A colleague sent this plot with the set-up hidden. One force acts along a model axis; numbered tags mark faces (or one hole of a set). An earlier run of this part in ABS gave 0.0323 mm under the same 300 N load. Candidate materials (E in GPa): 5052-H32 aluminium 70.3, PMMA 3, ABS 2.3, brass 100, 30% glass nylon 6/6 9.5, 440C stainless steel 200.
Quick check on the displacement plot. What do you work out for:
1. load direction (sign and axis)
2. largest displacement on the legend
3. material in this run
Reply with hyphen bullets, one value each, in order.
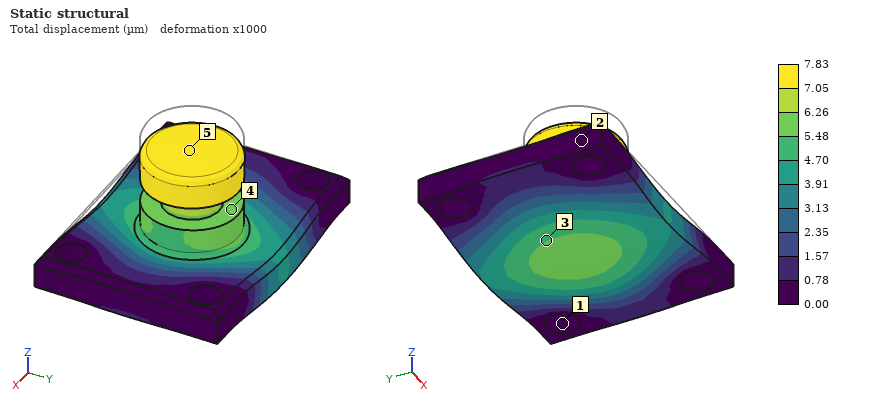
- -Z
- 7.83 µm
- 30% glass nylon 6/6
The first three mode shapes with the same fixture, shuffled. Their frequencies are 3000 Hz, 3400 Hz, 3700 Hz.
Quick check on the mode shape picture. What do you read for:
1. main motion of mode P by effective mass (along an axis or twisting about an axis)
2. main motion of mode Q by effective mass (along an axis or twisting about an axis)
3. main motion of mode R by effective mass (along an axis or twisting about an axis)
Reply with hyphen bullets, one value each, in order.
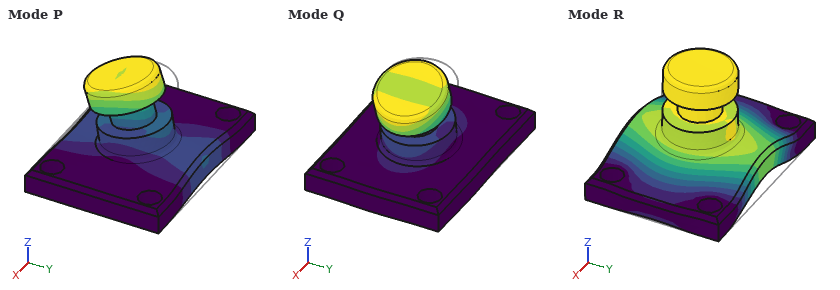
- along Y
- along X
- along Z
